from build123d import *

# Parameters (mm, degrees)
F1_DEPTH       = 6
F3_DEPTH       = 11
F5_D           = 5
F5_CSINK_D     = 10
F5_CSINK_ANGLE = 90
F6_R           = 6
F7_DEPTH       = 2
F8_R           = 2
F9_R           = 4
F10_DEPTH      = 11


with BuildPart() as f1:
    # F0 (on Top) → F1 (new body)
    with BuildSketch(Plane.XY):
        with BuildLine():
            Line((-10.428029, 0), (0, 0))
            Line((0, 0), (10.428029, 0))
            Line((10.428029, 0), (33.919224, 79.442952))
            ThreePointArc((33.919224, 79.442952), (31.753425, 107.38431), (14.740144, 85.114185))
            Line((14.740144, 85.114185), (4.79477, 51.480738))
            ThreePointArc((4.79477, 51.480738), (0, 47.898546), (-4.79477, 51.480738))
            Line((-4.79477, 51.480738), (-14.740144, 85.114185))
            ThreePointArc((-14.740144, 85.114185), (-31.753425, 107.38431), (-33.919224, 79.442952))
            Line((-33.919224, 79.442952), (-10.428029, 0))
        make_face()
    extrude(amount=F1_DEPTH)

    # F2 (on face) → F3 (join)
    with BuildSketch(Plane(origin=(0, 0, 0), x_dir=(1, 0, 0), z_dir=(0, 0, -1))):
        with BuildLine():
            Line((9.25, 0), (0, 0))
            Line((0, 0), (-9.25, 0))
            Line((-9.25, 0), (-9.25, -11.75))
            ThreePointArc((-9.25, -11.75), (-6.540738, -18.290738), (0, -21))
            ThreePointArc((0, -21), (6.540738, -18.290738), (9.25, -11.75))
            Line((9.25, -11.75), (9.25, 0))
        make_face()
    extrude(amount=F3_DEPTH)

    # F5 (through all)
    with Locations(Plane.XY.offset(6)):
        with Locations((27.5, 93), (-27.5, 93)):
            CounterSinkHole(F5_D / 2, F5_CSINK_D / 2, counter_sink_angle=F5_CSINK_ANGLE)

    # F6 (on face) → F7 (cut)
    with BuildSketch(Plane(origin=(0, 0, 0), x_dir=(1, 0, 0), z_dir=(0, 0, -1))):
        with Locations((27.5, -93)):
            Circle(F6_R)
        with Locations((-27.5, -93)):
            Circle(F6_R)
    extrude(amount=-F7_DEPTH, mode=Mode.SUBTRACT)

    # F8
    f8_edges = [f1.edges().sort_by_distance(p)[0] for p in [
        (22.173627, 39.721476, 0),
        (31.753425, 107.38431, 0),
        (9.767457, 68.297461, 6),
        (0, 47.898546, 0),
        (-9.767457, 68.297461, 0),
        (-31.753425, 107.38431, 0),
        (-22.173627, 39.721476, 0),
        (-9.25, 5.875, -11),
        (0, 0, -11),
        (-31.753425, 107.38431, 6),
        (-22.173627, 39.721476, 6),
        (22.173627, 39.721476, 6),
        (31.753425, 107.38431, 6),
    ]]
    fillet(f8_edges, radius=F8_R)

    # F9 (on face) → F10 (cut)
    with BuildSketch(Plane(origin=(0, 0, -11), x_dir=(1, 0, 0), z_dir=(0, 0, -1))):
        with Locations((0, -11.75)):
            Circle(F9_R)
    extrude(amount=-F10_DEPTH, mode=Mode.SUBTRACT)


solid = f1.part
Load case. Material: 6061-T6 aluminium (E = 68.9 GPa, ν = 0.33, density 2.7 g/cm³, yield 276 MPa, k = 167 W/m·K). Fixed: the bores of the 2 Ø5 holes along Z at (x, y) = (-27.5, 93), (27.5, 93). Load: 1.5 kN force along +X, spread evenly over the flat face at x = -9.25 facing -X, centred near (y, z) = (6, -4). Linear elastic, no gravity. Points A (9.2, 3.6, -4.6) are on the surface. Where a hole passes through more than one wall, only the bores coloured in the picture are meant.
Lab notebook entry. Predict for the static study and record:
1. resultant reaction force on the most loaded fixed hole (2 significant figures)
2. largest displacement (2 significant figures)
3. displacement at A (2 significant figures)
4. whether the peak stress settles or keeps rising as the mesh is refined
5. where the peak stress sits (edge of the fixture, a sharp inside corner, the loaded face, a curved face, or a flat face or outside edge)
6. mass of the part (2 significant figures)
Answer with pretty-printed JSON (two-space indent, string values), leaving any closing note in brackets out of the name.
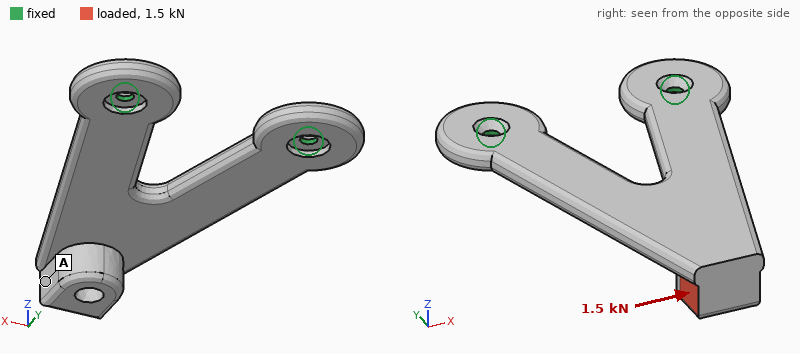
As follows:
{
  "resultant reaction force on the most loaded fixed hole": "2.4 kN",
  "largest displacement": "0.29 mm",
  "displacement at A": "0.22 mm",
  "whether the peak stress settles or keeps rising as the mesh is refined": "keeps rising",
  "where the peak stress sits": "edge of the fixture",
  "mass of the part": "77 g"
}
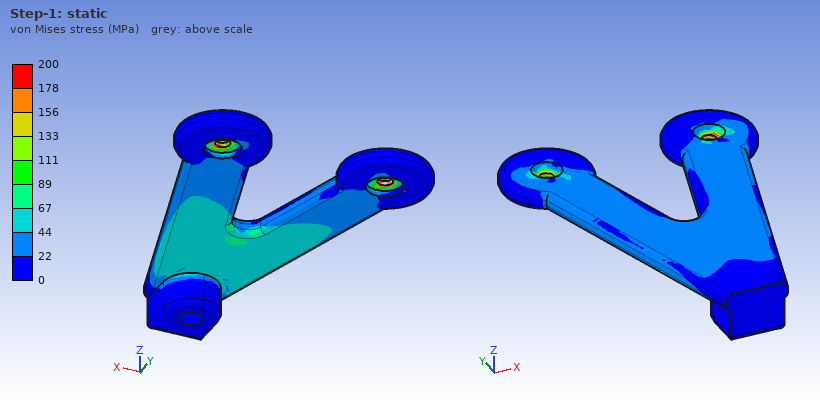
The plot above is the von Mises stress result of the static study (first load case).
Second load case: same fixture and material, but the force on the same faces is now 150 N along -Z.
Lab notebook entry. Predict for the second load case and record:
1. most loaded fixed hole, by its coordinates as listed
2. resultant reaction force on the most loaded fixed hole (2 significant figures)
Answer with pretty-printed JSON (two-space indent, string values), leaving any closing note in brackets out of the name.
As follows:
{
  "most loaded fixed hole, by its coordinates as listed": "(-27.5, 93)",
  "resultant reaction force on the most loaded fixed hole": "89 N"
}
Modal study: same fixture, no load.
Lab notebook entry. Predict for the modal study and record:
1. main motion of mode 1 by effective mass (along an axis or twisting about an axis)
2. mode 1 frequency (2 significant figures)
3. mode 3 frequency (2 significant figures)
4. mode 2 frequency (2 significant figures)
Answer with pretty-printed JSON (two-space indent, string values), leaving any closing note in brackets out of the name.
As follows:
{
  "main motion of mode 1 by effective mass": "along Z",
  "mode 1 frequency": "380 Hz",
  "mode 3 frequency": "2500 Hz",
  "mode 2 frequency": "2300 Hz"
}
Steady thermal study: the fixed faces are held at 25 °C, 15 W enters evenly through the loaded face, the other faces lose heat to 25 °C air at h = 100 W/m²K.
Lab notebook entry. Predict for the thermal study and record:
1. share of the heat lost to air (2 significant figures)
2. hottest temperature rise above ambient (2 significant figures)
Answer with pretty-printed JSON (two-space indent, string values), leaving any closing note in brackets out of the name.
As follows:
{
  "share of the heat lost to air": "62 %",
  "hottest temperature rise above ambient": "24 K"
}
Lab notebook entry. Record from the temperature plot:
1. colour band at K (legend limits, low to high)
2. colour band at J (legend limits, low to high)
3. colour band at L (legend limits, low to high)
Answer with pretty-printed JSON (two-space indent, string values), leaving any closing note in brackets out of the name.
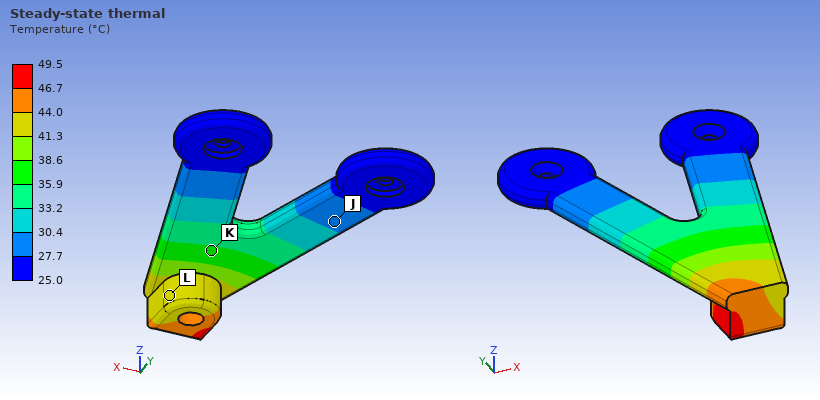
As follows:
{
  "colour band at K": "35.9 to 38.6 °C",
  "colour band at J": "27.7 to 30.4 °C",
  "colour band at L": "41.3 to 44.0 °C"
}
